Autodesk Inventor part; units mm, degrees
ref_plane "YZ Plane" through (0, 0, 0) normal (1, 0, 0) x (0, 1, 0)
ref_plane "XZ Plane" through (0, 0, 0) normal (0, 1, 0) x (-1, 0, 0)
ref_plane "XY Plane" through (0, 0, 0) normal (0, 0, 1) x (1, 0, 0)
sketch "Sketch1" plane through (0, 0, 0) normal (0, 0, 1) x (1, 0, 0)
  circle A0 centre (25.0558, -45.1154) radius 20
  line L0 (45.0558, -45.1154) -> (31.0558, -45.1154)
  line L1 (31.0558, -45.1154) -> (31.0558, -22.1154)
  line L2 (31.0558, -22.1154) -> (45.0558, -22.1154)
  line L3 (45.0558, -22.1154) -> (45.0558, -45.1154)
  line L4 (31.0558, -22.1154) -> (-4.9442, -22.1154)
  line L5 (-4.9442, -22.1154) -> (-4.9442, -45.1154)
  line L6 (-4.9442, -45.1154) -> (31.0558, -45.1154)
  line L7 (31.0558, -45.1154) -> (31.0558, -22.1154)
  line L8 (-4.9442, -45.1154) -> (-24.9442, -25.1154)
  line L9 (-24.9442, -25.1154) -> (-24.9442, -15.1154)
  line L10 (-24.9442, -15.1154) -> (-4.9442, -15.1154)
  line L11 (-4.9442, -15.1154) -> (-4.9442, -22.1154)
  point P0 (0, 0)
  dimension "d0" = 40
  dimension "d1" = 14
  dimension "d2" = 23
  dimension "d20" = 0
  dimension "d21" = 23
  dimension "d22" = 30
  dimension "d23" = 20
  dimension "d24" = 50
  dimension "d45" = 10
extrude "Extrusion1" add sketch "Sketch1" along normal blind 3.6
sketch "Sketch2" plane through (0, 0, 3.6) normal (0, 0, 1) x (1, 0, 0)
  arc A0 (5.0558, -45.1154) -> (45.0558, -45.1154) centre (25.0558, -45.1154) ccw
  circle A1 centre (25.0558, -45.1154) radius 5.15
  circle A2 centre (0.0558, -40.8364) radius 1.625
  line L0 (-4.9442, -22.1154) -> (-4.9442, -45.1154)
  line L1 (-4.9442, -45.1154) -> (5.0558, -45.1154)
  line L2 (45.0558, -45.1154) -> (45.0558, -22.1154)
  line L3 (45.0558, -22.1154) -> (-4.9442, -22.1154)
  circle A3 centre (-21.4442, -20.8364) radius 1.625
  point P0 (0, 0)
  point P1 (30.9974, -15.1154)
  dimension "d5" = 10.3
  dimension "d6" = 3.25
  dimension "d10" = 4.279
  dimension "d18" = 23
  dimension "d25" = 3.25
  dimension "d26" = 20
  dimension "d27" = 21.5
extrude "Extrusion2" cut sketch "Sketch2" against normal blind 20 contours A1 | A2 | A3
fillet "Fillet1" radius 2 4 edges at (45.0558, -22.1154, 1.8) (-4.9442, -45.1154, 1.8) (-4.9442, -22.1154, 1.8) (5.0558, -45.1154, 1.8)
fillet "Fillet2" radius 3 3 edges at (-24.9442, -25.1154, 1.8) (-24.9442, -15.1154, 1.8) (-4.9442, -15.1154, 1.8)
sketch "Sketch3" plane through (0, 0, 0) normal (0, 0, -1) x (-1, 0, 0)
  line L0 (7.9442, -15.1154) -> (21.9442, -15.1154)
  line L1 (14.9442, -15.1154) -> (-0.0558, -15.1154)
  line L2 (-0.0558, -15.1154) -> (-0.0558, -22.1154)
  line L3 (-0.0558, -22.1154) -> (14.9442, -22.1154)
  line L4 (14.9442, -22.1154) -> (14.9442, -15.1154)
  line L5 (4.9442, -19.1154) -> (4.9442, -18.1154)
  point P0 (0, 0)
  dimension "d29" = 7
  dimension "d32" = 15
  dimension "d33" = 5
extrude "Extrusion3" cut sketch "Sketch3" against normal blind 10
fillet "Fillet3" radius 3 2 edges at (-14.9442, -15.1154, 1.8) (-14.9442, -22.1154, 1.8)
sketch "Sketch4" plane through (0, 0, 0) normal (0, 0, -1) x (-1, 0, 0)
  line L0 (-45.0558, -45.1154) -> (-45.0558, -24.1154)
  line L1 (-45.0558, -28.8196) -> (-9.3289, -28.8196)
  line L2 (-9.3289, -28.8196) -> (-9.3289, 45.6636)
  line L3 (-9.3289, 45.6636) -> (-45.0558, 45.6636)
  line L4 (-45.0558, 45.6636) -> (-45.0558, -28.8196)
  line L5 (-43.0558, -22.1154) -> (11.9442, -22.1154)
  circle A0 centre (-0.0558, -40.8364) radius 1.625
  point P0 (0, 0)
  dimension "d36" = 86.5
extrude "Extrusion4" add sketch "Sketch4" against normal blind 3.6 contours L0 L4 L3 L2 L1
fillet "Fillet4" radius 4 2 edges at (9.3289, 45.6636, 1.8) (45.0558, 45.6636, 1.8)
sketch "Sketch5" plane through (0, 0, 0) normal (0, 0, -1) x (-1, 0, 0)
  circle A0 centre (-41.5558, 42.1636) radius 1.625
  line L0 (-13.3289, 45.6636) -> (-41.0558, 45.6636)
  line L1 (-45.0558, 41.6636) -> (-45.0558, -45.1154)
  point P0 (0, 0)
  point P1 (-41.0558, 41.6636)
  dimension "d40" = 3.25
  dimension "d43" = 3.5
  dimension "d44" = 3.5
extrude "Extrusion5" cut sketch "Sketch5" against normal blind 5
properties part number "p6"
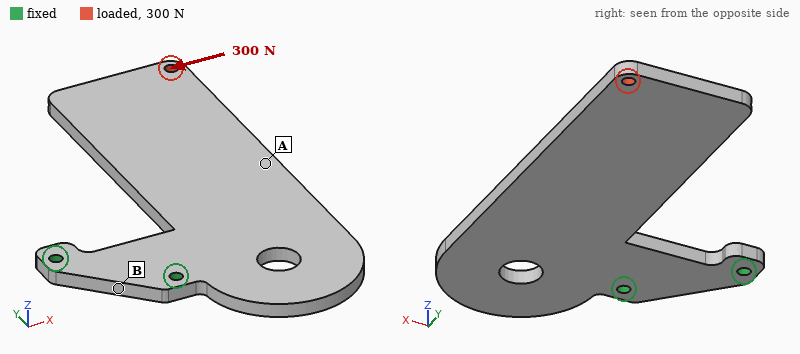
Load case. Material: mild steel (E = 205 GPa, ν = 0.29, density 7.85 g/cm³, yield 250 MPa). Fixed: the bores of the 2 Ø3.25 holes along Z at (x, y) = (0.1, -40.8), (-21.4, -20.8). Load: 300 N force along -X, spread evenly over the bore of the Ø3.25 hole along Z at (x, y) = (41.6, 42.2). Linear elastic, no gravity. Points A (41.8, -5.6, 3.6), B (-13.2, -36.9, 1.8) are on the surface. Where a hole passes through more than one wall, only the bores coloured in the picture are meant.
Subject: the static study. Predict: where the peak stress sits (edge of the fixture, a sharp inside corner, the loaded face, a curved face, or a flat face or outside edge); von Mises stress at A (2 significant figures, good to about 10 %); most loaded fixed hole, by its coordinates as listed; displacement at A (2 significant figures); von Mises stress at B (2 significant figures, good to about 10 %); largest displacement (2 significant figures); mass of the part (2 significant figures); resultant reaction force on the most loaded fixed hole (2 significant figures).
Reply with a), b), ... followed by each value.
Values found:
a) edge of the fixture
b) 16 MPa
c) (-21.4, -20.8)
d) 48 µm
e) 40 MPa
f) 99 µm
g) 120 g
h) 990 N
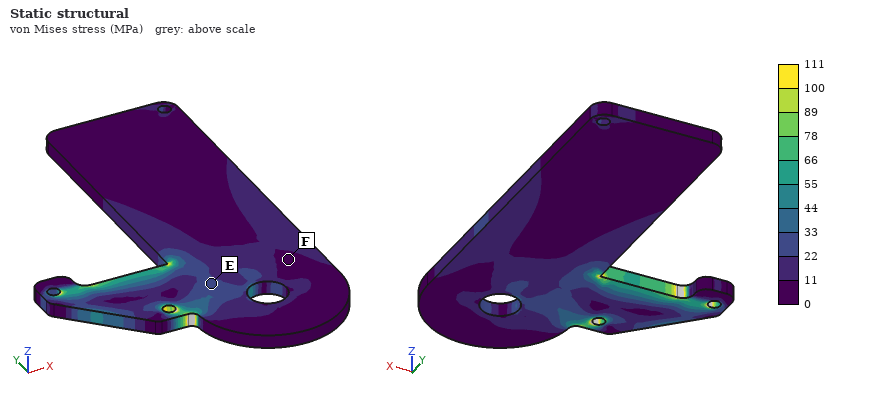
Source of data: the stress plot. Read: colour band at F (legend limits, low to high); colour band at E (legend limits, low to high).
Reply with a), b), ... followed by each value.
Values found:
a) 0 to 11 MPa
b) 22 to 33 MPa
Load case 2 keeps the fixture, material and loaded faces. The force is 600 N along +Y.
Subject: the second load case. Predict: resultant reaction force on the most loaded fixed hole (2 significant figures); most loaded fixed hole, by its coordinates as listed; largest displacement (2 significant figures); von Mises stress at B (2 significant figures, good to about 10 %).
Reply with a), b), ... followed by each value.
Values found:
a) 1.2 kN
b) (0.1, -40.8)
c) 90 µm
d) 37 MPa
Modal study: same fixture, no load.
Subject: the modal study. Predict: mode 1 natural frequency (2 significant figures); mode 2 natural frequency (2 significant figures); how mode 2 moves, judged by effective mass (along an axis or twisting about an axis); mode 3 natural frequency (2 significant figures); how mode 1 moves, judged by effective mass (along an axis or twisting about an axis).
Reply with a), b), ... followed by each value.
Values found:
a) 310 Hz
b) 940 Hz
c) along Z
d) 1500 Hz
e) along Z
